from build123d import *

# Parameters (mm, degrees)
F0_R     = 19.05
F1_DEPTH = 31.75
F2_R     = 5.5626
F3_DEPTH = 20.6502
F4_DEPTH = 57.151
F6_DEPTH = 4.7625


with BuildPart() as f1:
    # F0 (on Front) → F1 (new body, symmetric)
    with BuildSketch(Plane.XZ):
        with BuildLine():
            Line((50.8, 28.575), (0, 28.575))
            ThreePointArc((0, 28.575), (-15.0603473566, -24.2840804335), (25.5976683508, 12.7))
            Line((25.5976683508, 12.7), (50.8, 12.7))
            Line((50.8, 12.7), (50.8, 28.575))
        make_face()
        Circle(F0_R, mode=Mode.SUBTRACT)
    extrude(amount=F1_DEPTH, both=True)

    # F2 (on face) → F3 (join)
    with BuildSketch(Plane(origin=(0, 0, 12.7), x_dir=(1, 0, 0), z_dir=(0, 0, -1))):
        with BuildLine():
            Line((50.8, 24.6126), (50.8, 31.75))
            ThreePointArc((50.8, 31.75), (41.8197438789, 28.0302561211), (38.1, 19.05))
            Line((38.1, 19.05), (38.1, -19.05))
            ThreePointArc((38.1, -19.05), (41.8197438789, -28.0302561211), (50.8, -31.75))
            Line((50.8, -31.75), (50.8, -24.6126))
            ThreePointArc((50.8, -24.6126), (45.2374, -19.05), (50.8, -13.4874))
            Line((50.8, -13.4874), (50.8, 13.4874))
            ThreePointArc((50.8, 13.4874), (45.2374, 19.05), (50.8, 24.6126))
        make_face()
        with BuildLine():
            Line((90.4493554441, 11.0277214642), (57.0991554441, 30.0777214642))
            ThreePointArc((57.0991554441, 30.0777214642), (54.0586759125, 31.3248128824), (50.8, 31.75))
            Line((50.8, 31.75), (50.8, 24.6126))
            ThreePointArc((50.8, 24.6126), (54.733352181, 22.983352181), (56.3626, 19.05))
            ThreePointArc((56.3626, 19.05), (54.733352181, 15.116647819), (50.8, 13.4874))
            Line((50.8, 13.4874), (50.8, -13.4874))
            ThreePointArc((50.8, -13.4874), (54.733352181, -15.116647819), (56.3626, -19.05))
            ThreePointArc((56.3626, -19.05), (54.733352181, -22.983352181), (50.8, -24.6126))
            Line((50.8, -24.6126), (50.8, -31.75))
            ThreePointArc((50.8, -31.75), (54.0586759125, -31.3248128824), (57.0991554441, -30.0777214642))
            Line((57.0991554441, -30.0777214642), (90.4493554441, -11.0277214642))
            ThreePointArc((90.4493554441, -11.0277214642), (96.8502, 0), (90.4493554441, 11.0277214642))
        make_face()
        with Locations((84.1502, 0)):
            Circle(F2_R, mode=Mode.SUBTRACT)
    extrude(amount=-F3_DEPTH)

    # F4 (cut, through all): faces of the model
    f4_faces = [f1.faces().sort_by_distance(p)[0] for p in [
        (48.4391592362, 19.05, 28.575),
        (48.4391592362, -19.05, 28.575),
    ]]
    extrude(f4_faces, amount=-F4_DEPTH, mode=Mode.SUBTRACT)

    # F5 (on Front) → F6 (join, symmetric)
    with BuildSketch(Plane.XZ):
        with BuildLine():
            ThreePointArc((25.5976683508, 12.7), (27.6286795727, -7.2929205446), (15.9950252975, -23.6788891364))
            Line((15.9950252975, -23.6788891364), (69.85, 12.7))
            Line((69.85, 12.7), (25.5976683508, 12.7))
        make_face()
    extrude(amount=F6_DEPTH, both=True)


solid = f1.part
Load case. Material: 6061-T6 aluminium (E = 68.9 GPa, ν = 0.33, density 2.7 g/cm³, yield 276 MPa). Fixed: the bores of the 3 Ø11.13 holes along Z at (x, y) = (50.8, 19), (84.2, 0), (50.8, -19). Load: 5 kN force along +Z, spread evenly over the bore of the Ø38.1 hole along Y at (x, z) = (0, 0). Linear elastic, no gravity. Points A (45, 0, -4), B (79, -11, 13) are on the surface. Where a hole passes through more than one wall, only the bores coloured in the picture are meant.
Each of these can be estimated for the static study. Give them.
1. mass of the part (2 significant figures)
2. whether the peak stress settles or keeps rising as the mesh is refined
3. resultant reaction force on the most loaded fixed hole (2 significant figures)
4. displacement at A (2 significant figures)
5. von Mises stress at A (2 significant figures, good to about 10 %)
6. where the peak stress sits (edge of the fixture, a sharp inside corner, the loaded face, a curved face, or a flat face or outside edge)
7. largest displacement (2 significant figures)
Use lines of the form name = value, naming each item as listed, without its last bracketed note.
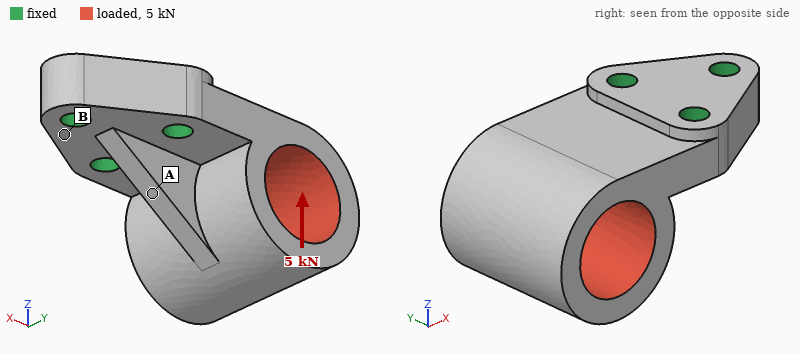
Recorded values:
mass of the part = 450 g
whether the peak stress settles or keeps rising as the mesh is refined = keeps rising
resultant reaction force on the most loaded fixed hole = 3.5 kN
displacement at A = 0.028 mm
von Mises stress at A = 39 MPa
where the peak stress sits = edge of the fixture
largest displacement = 0.14 mm
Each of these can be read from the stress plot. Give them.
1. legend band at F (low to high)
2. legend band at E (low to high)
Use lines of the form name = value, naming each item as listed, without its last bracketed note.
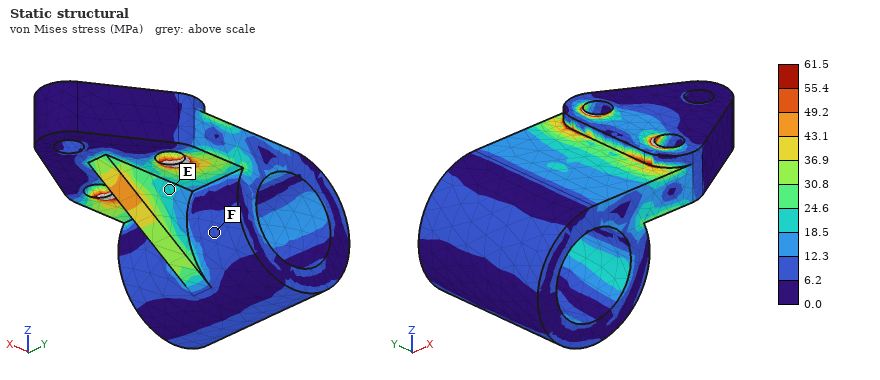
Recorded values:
legend band at F = 6.2 to 12.3 MPa
legend band at E = 18.5 to 24.6 MPa
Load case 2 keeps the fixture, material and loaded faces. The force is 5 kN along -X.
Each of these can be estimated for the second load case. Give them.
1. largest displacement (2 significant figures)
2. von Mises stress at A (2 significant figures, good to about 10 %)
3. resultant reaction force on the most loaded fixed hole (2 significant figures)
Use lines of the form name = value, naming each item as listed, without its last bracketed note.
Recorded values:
largest displacement = 71 µm
von Mises stress at A = 30 MPa
resultant reaction force on the most loaded fixed hole = 2.0 kN
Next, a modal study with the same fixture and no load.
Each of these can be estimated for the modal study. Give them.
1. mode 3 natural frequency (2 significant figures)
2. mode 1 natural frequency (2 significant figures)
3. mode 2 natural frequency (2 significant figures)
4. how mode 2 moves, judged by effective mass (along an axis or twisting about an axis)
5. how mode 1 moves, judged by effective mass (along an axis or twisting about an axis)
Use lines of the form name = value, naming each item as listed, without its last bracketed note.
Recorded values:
mode 3 natural frequency = 5900 Hz
mode 1 natural frequency = 2000 Hz
mode 2 natural frequency = 3300 Hz
how mode 2 moves, judged by effective mass = along Y
how mode 1 moves, judged by effective mass = along Z
